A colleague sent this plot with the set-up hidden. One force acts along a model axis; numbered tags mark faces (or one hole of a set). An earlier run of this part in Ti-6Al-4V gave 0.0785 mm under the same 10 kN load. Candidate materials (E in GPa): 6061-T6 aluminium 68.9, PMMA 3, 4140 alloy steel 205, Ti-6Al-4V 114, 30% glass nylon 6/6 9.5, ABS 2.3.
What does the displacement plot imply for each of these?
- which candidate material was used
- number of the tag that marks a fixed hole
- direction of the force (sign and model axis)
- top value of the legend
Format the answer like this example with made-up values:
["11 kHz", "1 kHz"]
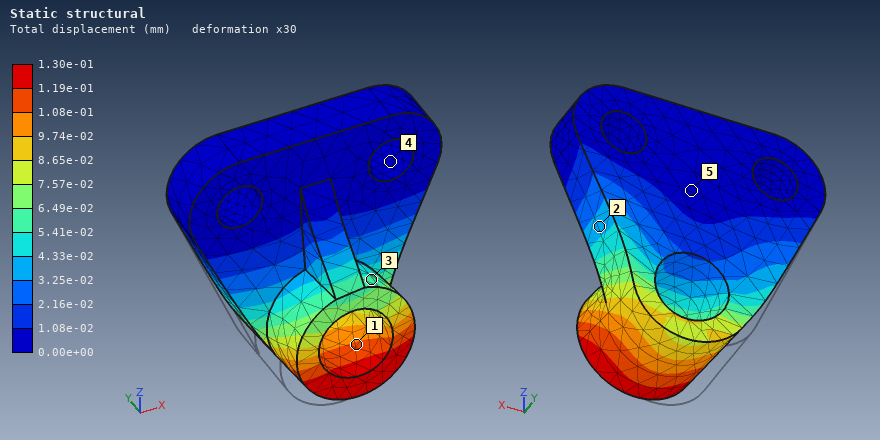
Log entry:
["6061-T6 aluminium", "4", "+X", "1.30e-01 mm"]
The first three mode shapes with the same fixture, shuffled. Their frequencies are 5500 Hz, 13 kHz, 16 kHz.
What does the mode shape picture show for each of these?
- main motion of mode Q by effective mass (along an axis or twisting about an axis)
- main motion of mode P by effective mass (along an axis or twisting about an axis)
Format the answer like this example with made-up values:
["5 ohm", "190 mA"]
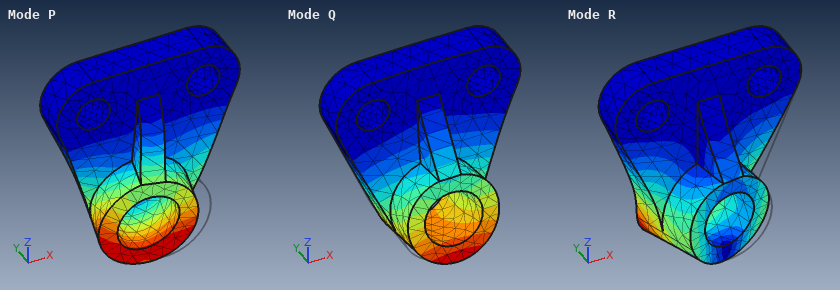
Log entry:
["along Y", "along X"]
